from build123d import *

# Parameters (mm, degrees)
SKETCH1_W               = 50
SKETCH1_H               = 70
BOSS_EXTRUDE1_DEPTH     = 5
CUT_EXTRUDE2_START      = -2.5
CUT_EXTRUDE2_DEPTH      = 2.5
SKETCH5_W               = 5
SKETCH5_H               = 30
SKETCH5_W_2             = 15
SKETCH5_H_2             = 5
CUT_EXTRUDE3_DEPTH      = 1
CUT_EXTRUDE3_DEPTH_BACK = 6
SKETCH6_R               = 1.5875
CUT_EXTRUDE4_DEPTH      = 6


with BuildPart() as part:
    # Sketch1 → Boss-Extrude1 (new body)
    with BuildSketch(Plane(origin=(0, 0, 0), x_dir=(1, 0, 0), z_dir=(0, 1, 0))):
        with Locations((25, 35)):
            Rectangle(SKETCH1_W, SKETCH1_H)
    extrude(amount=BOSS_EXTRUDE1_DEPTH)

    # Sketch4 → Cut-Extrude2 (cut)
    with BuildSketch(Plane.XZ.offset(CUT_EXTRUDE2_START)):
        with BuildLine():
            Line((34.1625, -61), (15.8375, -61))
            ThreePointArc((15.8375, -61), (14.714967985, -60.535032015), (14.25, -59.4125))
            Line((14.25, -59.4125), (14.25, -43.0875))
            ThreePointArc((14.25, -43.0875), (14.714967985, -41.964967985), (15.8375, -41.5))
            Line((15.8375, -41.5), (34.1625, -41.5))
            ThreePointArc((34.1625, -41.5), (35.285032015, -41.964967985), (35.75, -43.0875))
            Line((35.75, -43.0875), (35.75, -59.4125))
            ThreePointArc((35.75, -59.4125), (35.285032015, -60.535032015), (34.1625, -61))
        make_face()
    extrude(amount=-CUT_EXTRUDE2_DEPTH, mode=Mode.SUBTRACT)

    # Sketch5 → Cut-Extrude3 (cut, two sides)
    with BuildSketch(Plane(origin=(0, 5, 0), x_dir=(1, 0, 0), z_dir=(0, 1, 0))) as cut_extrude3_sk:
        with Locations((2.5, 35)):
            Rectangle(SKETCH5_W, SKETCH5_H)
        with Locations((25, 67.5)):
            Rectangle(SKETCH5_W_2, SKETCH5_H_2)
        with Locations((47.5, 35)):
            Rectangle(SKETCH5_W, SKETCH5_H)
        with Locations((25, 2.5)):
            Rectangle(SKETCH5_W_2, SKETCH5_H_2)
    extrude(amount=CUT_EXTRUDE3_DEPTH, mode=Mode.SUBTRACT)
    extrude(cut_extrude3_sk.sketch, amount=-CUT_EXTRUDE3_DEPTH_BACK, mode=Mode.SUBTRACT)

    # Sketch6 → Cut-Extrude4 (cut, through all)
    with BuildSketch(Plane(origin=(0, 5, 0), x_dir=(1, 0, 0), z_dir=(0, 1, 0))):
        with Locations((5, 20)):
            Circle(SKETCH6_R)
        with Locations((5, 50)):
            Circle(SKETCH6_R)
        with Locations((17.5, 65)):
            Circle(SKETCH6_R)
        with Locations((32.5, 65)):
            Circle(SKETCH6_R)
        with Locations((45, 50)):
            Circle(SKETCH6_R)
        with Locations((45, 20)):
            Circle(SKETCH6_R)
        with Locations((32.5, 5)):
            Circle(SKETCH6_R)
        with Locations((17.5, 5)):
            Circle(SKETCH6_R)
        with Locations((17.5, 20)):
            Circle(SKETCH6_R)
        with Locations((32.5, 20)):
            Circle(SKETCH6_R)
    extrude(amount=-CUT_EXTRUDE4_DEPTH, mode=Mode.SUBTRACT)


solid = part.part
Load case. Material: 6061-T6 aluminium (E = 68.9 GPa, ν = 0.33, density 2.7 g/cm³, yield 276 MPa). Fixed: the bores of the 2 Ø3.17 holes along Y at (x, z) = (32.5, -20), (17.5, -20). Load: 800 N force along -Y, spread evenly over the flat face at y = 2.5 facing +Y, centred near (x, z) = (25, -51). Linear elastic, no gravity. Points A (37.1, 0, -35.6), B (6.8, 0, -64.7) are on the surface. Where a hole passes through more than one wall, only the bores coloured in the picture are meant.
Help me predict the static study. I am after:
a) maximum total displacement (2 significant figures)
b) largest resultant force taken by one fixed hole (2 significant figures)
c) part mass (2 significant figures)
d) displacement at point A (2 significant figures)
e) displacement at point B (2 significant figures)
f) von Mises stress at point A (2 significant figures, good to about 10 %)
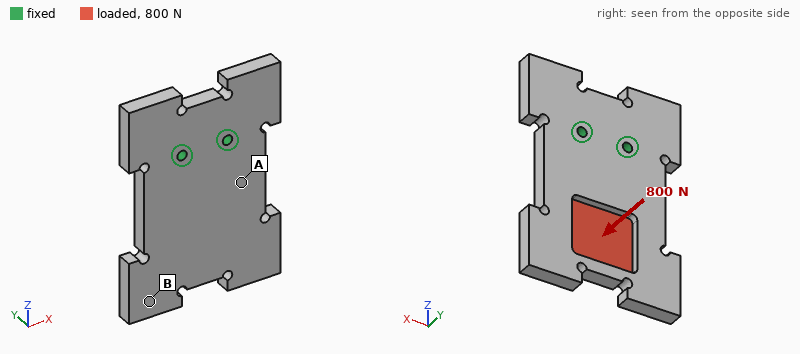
0.65 mm
400 N
38 g
0.11 mm
0.54 mm
74 MPa
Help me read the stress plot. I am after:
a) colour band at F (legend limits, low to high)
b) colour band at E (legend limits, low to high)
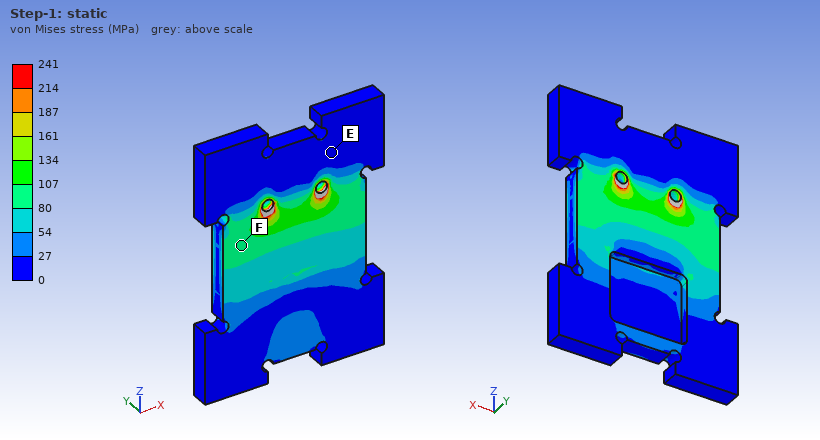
80 to 107 MPa
0 to 27 MPa
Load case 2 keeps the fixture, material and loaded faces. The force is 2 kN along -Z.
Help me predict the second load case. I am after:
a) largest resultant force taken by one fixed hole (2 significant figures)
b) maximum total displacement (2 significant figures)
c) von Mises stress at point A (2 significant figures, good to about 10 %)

1.0 kN
32 µm
9.0 MPa
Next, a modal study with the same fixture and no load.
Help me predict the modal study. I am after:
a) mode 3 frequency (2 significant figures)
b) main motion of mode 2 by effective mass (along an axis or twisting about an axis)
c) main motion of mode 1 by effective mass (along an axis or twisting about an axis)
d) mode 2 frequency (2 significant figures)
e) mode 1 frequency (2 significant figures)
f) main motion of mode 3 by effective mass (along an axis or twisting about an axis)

6200 Hz
twisting about Z
along Y
2600 Hz
1500 Hz
along X
